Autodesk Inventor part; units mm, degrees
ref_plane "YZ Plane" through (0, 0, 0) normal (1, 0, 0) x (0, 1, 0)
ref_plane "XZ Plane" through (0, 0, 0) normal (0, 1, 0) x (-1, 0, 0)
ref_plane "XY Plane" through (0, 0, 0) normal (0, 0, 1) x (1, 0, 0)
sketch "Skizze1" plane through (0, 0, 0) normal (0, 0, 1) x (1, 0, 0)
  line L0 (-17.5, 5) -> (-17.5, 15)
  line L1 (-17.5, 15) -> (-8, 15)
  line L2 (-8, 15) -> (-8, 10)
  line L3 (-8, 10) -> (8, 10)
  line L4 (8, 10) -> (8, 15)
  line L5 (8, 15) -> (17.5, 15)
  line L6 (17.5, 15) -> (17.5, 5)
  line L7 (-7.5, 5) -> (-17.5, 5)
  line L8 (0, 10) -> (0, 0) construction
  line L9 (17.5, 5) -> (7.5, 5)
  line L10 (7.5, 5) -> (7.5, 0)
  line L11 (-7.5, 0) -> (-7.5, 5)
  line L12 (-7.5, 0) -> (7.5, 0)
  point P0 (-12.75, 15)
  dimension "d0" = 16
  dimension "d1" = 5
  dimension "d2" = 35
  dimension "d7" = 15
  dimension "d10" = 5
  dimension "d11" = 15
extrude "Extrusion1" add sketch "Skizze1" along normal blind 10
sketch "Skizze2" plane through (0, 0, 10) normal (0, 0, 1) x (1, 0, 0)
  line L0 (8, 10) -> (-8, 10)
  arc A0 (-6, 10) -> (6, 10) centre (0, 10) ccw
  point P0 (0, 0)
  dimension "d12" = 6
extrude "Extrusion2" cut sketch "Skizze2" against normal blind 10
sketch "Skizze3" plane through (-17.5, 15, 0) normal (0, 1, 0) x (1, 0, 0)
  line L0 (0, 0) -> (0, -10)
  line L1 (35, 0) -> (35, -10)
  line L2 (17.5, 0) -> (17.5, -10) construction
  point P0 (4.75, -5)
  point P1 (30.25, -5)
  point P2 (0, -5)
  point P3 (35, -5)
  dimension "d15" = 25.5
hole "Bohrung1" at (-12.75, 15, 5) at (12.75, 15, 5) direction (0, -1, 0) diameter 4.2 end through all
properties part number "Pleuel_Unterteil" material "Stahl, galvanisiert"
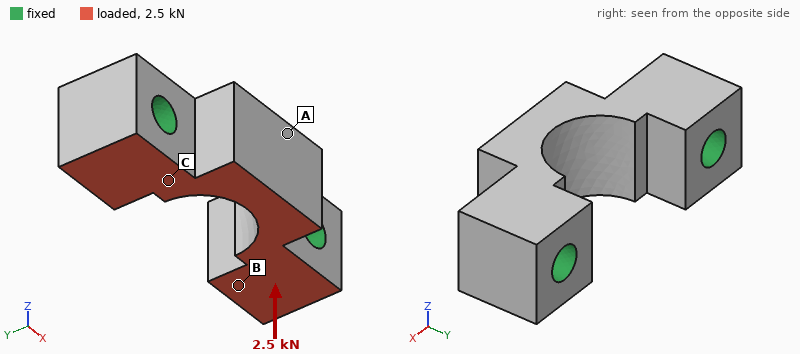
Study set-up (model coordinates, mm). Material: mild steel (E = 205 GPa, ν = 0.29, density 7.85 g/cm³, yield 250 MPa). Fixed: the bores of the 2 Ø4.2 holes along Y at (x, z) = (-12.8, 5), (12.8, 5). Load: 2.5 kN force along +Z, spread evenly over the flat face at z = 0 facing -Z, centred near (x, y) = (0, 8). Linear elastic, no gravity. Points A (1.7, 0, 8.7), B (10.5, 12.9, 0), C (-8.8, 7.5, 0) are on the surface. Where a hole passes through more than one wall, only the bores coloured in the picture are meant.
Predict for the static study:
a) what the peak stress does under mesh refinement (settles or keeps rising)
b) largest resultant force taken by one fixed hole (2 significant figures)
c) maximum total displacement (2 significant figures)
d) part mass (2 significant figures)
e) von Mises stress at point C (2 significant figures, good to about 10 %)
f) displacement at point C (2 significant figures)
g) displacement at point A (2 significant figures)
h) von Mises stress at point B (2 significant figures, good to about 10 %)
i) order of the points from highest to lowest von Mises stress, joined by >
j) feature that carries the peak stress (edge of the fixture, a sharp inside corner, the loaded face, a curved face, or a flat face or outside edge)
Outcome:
keeps rising
1.3 kN
4.3 µm
20 g
33 MPa
1.1 µm
3.8 µm
17 MPa
C > B > A
edge of the fixture
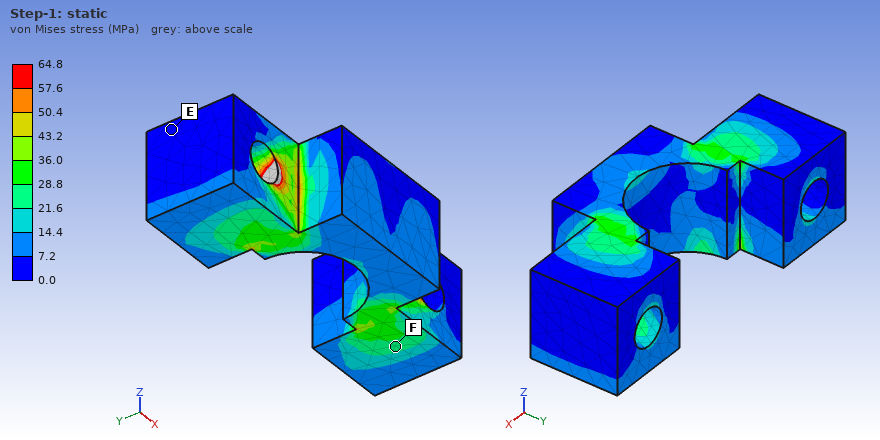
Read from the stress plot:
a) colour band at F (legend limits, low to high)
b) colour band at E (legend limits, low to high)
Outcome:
21.6 to 28.8 MPa
0.0 to 7.2 MPa
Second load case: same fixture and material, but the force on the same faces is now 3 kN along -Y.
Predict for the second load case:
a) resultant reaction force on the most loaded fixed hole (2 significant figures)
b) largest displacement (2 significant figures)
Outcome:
1.5 kN
6.2 µm
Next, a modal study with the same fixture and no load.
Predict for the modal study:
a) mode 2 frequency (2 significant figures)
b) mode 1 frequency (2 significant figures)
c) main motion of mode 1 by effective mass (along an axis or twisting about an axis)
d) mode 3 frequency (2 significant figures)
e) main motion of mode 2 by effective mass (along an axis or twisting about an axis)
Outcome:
57 kHz
31 kHz
along Z
61 kHz
along Y
